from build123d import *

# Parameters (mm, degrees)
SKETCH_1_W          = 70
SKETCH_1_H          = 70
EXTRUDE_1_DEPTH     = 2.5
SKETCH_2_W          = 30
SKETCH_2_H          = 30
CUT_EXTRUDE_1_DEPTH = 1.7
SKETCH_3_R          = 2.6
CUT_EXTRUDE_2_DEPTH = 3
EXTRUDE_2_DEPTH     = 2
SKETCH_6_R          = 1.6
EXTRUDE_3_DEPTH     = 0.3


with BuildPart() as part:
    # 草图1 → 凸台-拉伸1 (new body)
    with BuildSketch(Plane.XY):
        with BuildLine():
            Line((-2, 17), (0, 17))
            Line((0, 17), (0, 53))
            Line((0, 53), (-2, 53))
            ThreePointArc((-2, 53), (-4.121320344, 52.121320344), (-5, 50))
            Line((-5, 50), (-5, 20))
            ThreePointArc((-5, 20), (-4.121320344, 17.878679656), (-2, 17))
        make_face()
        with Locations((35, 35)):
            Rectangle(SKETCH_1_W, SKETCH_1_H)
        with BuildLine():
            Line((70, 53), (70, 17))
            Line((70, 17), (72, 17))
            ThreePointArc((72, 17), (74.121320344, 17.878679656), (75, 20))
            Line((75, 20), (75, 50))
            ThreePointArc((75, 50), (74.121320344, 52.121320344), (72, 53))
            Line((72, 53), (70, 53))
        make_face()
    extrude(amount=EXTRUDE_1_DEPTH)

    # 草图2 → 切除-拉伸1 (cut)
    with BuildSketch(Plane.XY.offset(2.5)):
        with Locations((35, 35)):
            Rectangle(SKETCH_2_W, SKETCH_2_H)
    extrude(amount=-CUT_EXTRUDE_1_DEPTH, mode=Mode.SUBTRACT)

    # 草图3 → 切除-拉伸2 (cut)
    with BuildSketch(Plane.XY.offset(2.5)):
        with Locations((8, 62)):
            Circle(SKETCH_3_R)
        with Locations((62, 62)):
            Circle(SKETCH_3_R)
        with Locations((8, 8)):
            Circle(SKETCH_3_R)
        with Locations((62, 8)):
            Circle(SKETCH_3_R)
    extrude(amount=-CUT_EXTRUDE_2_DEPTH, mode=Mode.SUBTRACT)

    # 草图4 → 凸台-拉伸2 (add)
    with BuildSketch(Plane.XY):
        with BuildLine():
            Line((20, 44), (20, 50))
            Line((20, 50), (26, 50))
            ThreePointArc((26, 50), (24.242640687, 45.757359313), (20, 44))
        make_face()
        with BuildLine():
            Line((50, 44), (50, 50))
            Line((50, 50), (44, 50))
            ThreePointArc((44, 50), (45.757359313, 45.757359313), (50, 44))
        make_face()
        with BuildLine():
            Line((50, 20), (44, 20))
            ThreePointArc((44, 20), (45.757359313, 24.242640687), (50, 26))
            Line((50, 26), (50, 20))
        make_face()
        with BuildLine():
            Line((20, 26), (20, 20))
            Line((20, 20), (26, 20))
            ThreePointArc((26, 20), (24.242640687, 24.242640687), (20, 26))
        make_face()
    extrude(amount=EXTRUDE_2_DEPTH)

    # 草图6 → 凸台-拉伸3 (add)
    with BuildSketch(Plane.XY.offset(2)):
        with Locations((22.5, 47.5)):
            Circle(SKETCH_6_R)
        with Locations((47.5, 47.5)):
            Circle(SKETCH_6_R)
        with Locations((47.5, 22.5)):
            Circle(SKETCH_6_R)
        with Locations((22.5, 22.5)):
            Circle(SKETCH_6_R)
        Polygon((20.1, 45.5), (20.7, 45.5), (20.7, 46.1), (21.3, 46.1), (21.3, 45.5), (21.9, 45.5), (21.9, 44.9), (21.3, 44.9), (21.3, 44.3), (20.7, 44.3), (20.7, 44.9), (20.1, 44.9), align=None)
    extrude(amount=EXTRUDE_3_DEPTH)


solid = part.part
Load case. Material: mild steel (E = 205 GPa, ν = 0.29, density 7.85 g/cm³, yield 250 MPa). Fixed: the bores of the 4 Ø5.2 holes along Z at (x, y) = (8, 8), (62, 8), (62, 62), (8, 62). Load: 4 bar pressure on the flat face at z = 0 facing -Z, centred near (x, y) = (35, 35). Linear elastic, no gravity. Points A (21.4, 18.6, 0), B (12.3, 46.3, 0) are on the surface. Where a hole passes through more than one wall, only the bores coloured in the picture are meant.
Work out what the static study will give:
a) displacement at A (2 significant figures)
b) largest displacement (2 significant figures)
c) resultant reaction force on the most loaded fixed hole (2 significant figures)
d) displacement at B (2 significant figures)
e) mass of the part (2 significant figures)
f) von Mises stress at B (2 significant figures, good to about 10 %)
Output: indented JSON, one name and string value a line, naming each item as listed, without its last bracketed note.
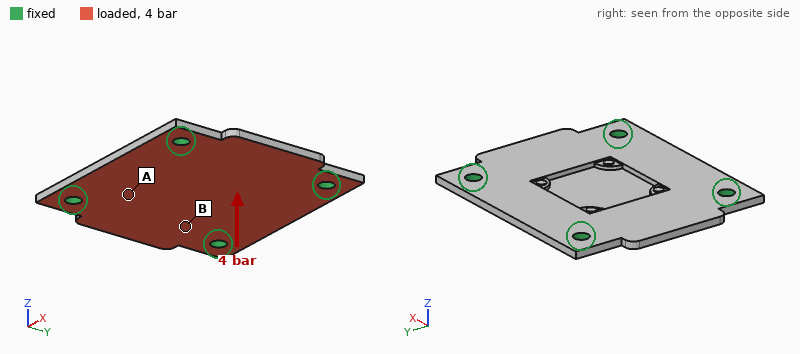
{
  "displacement at A": "0.045 mm",
  "largest displacement": "0.13 mm",
  "resultant reaction force on the most loaded fixed hole": "600 N",
  "displacement at B": "0.037 mm",
  "mass of the part": "91 g",
  "von Mises stress at B": "42 MPa"
}
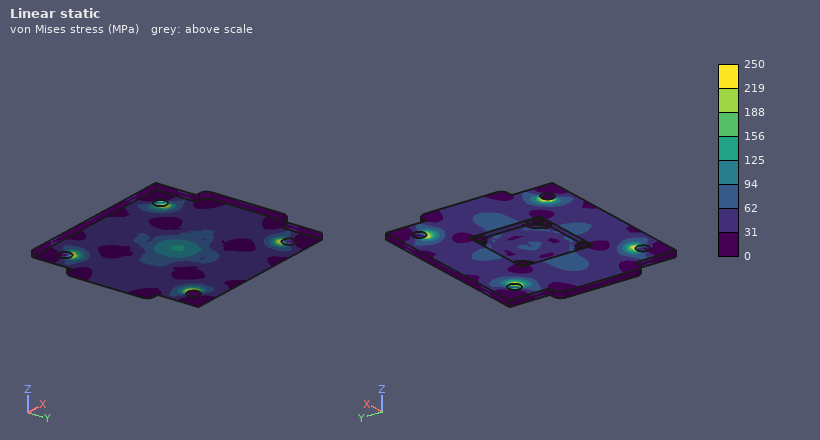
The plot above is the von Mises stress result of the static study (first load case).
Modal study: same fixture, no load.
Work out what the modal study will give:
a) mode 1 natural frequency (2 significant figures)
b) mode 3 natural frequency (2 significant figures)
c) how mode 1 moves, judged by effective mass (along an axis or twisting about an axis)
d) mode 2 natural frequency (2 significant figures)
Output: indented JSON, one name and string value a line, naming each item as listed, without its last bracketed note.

{
  "mode 1 natural frequency": "3700 Hz",
  "mode 3 natural frequency": "4600 Hz",
  "how mode 1 moves, judged by effective mass": "along Z",
  "mode 2 natural frequency": "4500 Hz"
}
